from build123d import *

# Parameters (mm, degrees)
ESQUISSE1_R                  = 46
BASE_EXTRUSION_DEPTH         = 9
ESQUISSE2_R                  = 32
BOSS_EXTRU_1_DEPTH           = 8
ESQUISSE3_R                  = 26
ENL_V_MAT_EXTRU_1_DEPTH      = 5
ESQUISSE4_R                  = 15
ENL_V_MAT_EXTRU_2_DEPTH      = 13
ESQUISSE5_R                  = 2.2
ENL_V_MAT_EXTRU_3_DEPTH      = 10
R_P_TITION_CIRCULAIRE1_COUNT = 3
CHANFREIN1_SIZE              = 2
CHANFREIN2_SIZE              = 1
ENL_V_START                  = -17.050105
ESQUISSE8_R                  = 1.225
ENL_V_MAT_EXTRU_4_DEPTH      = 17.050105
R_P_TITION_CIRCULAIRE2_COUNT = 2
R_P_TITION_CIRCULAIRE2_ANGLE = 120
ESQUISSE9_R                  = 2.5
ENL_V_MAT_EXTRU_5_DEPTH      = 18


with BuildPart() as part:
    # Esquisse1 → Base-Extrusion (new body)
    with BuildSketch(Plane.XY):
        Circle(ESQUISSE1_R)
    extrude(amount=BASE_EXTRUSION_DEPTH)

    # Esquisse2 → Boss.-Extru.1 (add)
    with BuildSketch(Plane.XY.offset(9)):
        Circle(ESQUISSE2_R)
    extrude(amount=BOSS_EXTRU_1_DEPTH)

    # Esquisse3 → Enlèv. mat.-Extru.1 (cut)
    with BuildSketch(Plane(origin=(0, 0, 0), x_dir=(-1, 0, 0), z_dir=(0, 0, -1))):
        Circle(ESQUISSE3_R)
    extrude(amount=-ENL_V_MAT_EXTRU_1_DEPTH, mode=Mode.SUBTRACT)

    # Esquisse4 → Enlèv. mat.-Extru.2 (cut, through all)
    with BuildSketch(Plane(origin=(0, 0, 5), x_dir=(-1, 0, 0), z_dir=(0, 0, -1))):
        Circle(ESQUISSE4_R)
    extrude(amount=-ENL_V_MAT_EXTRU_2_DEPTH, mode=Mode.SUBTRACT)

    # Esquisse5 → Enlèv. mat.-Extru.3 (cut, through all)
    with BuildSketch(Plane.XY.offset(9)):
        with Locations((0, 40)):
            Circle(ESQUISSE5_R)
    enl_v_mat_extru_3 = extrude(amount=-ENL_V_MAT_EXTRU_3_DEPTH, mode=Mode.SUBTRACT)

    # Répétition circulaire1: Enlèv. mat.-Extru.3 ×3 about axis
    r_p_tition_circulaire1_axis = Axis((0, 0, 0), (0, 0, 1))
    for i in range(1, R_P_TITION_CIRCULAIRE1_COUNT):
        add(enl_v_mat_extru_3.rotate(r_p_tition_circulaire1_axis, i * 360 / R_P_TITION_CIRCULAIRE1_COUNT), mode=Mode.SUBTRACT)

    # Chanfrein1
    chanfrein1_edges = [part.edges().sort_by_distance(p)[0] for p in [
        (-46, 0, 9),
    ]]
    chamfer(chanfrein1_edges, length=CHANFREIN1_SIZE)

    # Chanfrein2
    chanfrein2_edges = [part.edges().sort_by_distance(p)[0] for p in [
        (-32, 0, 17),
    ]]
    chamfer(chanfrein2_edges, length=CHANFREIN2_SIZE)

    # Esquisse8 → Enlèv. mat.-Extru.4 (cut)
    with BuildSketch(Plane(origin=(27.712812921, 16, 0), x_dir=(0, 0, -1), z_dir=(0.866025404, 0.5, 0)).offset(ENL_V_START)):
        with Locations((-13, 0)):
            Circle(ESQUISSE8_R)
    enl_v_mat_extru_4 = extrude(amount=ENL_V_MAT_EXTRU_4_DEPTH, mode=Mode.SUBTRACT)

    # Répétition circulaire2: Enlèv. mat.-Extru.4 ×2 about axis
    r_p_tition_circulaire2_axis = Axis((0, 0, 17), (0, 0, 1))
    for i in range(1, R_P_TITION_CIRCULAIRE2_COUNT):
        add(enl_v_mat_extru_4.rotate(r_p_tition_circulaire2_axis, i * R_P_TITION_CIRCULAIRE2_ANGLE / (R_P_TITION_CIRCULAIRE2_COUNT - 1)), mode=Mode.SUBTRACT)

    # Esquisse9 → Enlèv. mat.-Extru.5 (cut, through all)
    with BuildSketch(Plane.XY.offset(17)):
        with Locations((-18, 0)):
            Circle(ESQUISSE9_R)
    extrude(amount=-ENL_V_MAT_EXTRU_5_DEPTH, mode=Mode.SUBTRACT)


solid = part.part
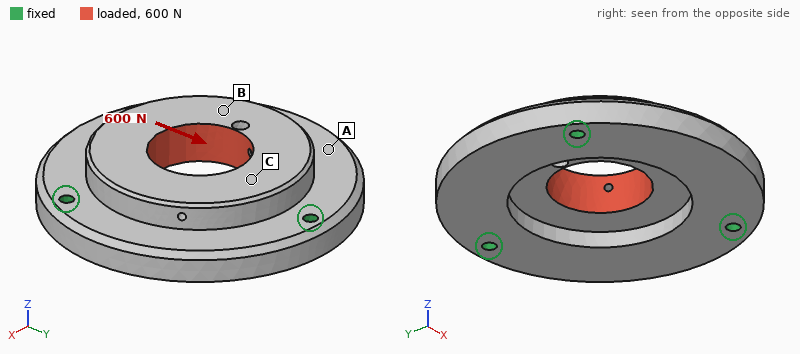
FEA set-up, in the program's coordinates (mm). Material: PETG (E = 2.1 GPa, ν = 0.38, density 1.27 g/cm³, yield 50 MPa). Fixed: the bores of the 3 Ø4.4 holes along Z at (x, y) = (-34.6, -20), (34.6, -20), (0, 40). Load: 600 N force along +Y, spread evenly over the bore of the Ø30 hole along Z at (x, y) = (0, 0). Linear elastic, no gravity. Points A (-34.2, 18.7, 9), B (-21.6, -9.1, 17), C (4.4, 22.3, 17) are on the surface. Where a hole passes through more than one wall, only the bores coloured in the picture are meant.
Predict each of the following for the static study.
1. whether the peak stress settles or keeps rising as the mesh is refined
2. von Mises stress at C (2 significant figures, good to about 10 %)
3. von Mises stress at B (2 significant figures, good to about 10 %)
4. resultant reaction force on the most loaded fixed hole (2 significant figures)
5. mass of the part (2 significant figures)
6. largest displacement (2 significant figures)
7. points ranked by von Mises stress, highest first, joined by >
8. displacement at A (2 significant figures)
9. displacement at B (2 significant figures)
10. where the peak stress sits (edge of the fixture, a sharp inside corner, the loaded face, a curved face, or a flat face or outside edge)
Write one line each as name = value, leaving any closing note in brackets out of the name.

whether the peak stress settles or keeps rising as the mesh is refined = keeps rising
von Mises stress at C = 1.0 MPa
von Mises stress at B = 0.66 MPa
resultant reaction force on the most loaded fixed hole = 210 N
mass of the part = 83 g
largest displacement = 37 µm
points ranked by von Mises stress, highest first, joined by > = C > B > A
displacement at A = 17 µm
displacement at B = 20 µm
where the peak stress sits = edge of the fixture
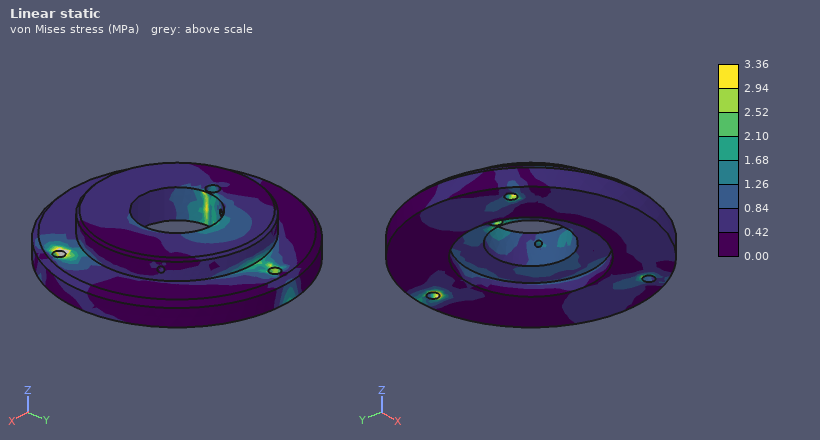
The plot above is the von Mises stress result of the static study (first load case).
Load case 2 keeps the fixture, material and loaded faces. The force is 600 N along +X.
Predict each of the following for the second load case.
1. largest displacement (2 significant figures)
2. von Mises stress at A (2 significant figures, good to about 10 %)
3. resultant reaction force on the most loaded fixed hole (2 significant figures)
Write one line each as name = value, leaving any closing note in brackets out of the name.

largest displacement = 36 µm
von Mises stress at A = 0.38 MPa
resultant reaction force on the most loaded fixed hole = 210 N
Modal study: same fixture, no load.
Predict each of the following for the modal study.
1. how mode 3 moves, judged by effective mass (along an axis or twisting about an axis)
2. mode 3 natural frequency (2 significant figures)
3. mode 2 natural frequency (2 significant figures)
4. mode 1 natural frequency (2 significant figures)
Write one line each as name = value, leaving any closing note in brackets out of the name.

how mode 3 moves, judged by effective mass = along Z
mode 3 natural frequency = 2000 Hz
mode 2 natural frequency = 1700 Hz
mode 1 natural frequency = 1700 Hz
